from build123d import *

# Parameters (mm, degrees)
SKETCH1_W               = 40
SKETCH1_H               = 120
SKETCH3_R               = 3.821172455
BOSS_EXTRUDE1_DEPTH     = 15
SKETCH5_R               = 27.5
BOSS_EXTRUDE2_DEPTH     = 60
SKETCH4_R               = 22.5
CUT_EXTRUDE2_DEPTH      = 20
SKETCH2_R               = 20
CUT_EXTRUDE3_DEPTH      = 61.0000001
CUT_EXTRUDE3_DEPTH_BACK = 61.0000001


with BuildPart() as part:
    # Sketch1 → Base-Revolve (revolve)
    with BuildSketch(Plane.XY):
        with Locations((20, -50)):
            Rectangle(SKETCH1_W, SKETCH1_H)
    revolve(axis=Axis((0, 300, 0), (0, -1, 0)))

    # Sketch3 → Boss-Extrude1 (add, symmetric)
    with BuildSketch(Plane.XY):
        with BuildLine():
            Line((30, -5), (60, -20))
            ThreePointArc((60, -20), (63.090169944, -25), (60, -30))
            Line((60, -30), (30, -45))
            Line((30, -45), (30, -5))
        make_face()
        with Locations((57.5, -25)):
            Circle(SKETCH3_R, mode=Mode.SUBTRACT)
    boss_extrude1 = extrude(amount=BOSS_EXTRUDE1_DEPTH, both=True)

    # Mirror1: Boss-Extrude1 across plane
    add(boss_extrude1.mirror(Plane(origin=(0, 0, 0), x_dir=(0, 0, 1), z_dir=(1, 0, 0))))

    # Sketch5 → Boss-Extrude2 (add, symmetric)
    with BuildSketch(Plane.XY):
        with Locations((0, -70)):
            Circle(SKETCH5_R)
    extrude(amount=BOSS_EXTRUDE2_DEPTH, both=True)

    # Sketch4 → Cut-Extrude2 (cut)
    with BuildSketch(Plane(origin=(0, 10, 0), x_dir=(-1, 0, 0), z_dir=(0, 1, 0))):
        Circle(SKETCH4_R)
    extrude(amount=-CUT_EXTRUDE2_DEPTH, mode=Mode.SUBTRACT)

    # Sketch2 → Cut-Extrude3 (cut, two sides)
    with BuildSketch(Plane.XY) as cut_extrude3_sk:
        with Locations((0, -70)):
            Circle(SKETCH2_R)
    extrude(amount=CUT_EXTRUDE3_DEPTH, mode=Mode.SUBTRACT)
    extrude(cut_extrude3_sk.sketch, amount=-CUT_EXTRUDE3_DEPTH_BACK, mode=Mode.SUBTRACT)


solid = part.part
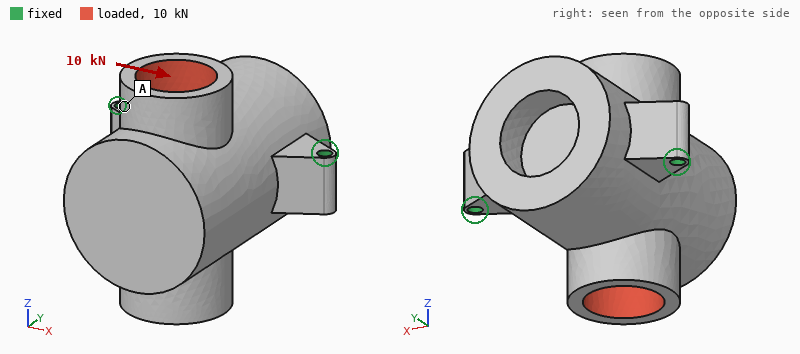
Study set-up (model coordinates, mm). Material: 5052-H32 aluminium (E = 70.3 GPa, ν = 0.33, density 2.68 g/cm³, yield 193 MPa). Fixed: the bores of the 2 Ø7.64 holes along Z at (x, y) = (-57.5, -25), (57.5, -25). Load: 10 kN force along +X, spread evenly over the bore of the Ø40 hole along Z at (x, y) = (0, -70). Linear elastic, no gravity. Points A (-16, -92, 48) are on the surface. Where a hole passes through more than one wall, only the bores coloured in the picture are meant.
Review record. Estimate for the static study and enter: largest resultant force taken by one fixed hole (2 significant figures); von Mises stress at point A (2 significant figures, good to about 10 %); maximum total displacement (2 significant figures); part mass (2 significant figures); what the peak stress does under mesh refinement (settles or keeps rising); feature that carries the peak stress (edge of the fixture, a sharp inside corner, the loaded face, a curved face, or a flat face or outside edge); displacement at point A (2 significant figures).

6.5 kN
3.9 MPa
29 µm
1.5 kg
keeps rising
edge of the fixture
25 µm
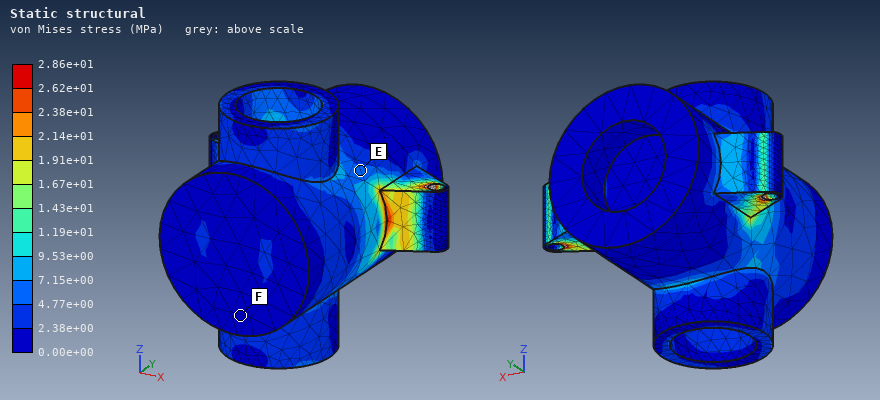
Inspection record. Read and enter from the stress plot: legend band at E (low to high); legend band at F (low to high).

4.77e+00 to 7.15e+00 MPa
0.00e+00 to 2.38e+00 MPa
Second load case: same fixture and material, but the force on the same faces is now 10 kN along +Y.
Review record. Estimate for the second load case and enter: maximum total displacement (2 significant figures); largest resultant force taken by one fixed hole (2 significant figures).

16 µm
5.1 kN
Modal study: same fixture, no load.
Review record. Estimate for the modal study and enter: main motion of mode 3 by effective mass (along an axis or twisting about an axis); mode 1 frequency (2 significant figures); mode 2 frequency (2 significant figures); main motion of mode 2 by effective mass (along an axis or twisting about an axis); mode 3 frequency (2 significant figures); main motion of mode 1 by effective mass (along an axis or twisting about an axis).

along Y
1100 Hz
3400 Hz
along X
3900 Hz
along Z
